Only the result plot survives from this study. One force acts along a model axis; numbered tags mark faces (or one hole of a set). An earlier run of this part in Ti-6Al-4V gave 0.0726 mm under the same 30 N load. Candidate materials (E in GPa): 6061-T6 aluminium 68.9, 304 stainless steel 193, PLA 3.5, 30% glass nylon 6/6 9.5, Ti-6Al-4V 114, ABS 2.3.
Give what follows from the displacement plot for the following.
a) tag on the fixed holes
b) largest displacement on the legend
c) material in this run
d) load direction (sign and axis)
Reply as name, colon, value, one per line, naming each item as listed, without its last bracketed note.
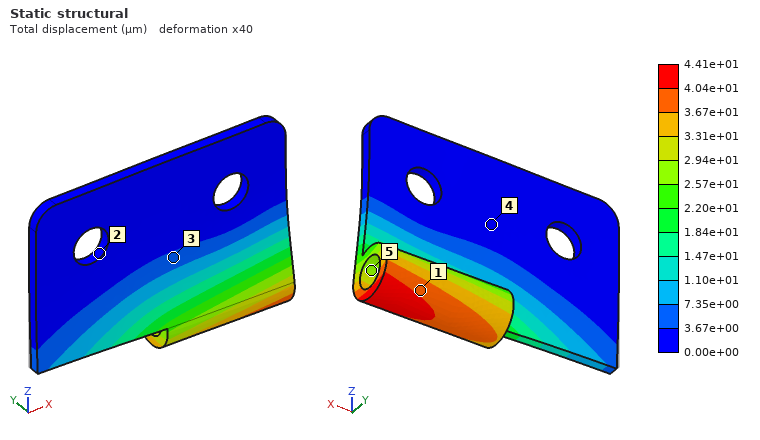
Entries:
tag on the fixed holes: 2
largest displacement on the legend: 4.41e+01 µm
material in this run: 304 stainless steel
load direction: -Y
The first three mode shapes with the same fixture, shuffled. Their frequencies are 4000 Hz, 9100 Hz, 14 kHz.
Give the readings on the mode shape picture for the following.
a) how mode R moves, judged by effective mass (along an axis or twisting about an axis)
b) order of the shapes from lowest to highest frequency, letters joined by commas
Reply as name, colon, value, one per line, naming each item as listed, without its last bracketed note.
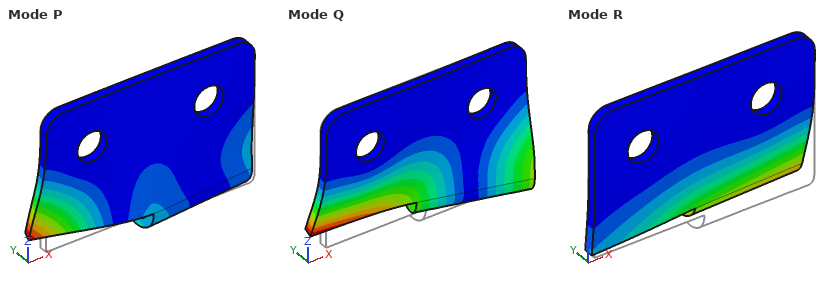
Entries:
how mode R moves, judged by effective mass: along Y
order of the shapes from lowest to highest frequency, letters joined by commas: R, Q, P
